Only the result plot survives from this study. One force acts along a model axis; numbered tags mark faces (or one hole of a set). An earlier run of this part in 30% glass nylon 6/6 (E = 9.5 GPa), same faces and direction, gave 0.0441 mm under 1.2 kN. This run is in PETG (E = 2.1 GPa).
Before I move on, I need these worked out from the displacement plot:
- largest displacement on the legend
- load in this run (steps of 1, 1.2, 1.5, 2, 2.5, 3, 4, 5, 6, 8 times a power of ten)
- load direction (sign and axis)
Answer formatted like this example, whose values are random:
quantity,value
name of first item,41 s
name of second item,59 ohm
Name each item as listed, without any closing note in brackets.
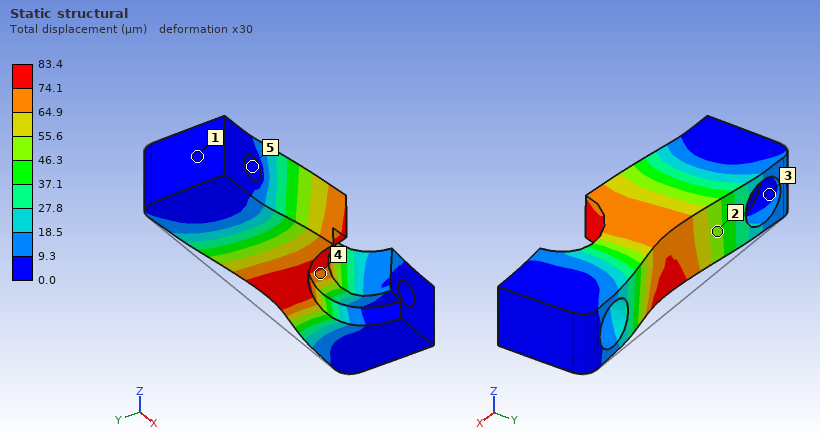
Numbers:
quantity,value
largest displacement on the legend,83.4 µm
load in this run,500 N
load direction,-Y
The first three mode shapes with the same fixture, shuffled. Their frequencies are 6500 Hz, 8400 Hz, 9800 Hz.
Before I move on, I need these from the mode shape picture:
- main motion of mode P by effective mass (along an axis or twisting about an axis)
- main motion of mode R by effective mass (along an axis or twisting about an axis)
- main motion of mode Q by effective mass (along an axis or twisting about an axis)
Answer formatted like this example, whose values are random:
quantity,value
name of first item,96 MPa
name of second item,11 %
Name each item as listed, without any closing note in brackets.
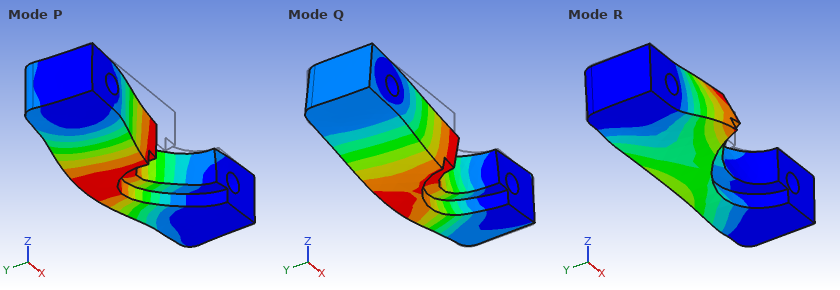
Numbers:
quantity,value
main motion of mode P by effective mass,along Y
main motion of mode R by effective mass,twisting about X
main motion of mode Q by effective mass,along Z
